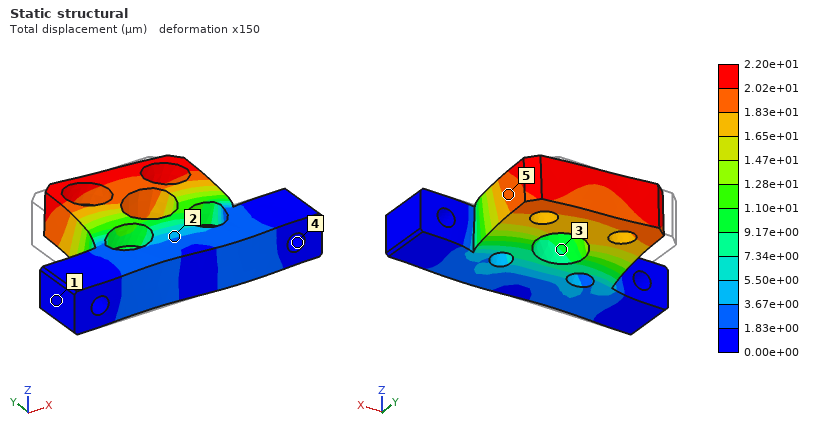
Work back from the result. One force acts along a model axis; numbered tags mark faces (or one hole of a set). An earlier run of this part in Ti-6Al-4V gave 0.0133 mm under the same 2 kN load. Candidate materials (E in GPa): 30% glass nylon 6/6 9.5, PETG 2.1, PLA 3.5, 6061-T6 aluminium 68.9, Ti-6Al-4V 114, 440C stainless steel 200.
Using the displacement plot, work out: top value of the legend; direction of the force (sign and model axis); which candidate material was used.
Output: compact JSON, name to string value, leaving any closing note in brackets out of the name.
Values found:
{"top value of the legend": "2.20e+01 µm", "direction of the force": "+X", "which candidate material was used": "6061-T6 aluminium"}
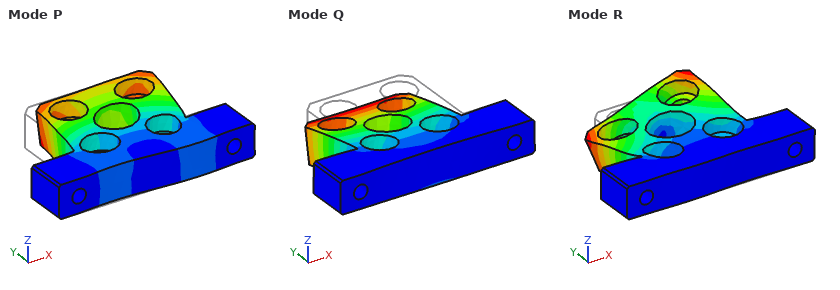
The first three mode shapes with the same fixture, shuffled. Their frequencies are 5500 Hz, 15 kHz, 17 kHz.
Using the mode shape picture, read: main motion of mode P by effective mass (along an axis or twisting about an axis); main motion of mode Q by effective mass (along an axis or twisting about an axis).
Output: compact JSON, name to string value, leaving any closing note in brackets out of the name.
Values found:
{"main motion of mode P by effective mass": "along X", "main motion of mode Q by effective mass": "along Z"}
